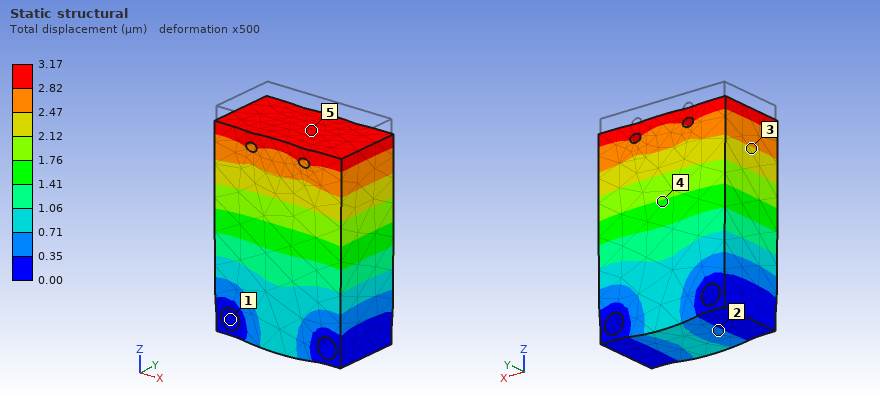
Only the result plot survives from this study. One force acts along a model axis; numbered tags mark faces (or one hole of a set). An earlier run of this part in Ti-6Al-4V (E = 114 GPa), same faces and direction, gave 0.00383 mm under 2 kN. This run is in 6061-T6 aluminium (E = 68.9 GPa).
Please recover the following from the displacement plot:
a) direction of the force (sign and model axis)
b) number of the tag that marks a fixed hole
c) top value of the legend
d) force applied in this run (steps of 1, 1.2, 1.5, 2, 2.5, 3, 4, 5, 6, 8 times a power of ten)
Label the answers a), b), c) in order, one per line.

a) -Z
b) 1
c) 3.17 µm
d) 1 kN
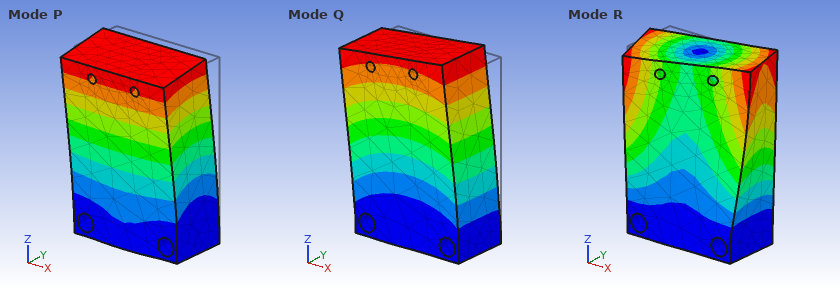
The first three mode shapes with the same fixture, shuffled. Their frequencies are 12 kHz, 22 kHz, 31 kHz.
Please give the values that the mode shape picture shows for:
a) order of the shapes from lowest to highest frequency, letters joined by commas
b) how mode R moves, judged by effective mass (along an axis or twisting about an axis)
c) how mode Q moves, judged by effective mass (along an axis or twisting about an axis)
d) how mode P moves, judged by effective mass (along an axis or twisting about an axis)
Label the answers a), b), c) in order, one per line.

a) P, Q, R
b) twisting about Z
c) along X
d) along Y
